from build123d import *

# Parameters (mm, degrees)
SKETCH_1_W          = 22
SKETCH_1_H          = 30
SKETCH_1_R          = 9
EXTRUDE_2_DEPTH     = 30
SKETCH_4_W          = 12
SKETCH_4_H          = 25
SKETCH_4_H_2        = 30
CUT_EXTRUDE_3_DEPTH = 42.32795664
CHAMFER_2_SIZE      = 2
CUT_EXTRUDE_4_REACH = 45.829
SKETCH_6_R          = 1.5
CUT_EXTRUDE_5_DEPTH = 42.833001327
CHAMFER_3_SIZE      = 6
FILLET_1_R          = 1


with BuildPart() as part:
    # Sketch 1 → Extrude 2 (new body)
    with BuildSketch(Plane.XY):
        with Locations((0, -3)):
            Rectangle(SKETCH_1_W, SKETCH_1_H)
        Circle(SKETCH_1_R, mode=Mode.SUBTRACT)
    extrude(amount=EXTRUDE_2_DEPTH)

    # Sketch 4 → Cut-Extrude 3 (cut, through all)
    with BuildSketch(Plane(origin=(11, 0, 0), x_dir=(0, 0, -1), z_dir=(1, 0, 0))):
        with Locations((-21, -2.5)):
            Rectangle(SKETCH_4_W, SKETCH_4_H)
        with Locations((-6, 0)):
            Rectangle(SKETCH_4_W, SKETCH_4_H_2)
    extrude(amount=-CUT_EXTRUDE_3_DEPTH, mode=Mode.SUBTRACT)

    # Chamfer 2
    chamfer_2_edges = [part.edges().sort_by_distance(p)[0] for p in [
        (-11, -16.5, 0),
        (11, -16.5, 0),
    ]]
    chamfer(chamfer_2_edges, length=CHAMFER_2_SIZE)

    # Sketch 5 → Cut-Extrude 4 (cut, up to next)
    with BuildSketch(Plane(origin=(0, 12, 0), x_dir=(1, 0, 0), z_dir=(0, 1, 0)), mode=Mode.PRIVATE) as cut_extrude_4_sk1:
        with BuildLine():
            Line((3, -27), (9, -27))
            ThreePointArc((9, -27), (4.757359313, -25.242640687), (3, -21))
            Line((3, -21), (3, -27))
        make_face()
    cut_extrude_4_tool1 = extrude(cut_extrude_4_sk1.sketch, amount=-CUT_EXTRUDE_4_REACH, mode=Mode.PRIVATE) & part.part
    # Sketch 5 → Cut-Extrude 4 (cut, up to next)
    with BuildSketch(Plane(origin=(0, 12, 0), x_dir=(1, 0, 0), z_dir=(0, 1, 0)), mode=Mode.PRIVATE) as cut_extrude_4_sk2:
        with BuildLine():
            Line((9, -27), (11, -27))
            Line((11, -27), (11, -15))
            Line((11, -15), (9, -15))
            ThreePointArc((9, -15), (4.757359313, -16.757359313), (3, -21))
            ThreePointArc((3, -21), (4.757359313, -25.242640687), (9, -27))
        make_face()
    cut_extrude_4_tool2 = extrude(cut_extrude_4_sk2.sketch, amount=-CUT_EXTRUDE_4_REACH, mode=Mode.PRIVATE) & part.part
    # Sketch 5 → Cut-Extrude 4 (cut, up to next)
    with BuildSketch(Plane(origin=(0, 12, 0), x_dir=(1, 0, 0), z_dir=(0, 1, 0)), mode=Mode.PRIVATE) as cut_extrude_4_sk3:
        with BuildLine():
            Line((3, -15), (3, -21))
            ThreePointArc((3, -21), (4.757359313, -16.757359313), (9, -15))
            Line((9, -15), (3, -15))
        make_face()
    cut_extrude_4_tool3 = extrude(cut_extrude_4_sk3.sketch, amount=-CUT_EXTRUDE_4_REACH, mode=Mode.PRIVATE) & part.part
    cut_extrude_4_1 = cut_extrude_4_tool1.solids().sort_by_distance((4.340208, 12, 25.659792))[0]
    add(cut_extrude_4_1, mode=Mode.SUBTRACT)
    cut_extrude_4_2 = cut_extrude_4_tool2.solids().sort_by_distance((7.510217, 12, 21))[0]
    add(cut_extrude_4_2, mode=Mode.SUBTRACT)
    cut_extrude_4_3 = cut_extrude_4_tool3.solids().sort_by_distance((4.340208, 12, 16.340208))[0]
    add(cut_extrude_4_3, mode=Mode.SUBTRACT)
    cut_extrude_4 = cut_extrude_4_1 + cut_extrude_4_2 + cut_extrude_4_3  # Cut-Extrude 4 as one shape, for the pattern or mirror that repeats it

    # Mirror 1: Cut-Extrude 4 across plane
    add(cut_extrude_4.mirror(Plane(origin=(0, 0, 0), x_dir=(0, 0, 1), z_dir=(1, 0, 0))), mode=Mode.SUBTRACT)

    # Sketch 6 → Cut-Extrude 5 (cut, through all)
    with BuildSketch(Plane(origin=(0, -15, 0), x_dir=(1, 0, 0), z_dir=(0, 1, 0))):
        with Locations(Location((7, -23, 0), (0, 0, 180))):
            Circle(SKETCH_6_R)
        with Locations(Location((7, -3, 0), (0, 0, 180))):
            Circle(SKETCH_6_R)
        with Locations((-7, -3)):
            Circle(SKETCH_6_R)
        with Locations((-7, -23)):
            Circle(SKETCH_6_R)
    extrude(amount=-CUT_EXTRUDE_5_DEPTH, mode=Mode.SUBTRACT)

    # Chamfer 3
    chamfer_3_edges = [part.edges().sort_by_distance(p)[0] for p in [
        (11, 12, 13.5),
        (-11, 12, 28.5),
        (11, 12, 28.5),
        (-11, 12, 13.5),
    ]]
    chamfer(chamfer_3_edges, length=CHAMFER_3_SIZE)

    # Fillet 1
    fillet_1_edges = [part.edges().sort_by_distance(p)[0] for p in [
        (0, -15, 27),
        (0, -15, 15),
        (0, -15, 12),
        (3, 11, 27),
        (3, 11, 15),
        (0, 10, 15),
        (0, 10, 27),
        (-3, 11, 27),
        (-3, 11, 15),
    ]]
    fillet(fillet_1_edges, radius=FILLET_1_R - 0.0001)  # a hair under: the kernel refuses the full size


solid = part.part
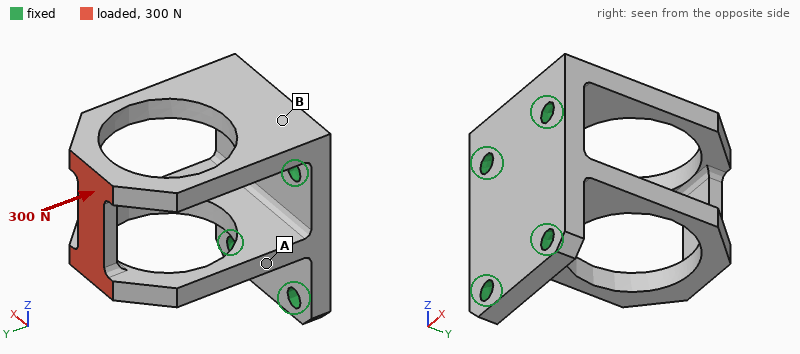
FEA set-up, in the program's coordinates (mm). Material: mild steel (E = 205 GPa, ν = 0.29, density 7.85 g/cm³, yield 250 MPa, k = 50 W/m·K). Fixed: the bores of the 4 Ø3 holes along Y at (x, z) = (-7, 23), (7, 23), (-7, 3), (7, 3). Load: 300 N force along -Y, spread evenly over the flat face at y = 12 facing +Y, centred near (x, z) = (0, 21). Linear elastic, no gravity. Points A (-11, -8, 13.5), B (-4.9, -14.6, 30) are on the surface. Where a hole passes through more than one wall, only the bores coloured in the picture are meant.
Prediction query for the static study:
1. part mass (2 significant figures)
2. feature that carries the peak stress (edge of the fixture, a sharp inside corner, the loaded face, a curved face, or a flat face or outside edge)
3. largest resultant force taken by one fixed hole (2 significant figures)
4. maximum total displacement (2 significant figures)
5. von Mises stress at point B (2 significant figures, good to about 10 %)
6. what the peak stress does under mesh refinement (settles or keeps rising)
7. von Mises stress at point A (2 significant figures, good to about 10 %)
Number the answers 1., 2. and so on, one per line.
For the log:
1. 30 g
2. a sharp inside corner
3. 120 N
4. 11 µm
5. 7.5 MPa
6. keeps rising
7. 23 MPa
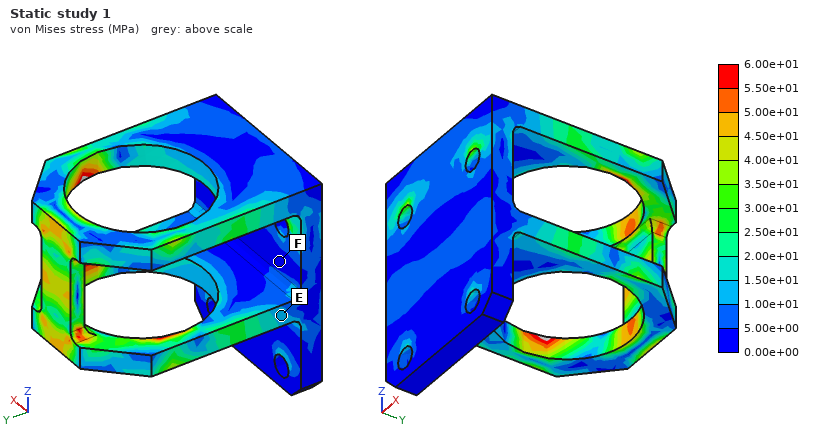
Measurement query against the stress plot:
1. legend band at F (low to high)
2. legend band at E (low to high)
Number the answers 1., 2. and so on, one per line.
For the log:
1. 0.00e+00 to 5.00e+00 MPa
2. 1.00e+01 to 1.50e+01 MPa
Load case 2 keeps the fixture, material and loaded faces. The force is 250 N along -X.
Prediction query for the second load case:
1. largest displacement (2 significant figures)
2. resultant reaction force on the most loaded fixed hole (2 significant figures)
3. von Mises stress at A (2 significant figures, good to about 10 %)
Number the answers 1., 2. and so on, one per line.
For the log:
1. 27 µm
2. 350 N
3. 50 MPa
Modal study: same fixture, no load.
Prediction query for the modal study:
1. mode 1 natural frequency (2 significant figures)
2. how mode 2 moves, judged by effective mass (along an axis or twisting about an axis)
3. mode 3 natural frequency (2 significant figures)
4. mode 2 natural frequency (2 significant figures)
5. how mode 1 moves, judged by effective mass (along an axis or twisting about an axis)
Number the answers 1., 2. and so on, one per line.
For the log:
1. 3600 Hz
2. along X
3. 8000 Hz
4. 6700 Hz
5. along Z
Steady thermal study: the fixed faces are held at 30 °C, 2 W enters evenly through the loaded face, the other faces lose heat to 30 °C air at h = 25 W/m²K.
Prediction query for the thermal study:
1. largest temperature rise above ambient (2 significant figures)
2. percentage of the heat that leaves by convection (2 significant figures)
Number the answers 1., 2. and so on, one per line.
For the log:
1. 28 K
2. 27 %
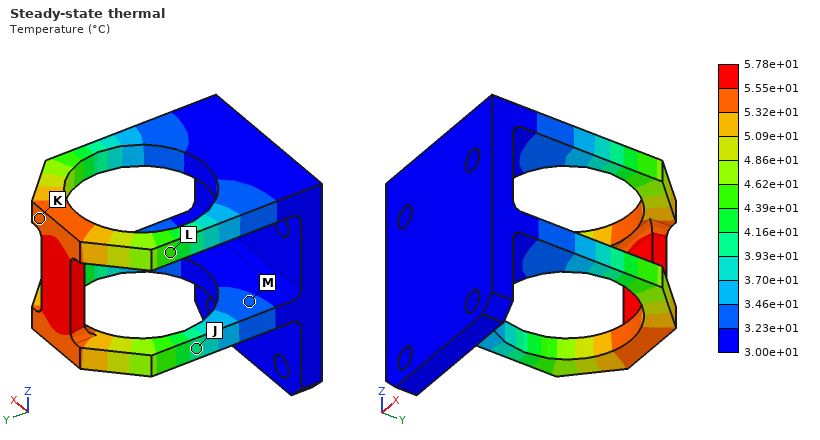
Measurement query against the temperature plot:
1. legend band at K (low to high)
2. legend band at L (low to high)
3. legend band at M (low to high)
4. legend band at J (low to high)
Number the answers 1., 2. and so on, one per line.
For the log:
1. 5.32e+01 to 5.55e+01 °C
2. 4.39e+01 to 4.62e+01 °C
3. 3.23e+01 to 3.46e+01 °C
4. 3.93e+01 to 4.16e+01 °C
